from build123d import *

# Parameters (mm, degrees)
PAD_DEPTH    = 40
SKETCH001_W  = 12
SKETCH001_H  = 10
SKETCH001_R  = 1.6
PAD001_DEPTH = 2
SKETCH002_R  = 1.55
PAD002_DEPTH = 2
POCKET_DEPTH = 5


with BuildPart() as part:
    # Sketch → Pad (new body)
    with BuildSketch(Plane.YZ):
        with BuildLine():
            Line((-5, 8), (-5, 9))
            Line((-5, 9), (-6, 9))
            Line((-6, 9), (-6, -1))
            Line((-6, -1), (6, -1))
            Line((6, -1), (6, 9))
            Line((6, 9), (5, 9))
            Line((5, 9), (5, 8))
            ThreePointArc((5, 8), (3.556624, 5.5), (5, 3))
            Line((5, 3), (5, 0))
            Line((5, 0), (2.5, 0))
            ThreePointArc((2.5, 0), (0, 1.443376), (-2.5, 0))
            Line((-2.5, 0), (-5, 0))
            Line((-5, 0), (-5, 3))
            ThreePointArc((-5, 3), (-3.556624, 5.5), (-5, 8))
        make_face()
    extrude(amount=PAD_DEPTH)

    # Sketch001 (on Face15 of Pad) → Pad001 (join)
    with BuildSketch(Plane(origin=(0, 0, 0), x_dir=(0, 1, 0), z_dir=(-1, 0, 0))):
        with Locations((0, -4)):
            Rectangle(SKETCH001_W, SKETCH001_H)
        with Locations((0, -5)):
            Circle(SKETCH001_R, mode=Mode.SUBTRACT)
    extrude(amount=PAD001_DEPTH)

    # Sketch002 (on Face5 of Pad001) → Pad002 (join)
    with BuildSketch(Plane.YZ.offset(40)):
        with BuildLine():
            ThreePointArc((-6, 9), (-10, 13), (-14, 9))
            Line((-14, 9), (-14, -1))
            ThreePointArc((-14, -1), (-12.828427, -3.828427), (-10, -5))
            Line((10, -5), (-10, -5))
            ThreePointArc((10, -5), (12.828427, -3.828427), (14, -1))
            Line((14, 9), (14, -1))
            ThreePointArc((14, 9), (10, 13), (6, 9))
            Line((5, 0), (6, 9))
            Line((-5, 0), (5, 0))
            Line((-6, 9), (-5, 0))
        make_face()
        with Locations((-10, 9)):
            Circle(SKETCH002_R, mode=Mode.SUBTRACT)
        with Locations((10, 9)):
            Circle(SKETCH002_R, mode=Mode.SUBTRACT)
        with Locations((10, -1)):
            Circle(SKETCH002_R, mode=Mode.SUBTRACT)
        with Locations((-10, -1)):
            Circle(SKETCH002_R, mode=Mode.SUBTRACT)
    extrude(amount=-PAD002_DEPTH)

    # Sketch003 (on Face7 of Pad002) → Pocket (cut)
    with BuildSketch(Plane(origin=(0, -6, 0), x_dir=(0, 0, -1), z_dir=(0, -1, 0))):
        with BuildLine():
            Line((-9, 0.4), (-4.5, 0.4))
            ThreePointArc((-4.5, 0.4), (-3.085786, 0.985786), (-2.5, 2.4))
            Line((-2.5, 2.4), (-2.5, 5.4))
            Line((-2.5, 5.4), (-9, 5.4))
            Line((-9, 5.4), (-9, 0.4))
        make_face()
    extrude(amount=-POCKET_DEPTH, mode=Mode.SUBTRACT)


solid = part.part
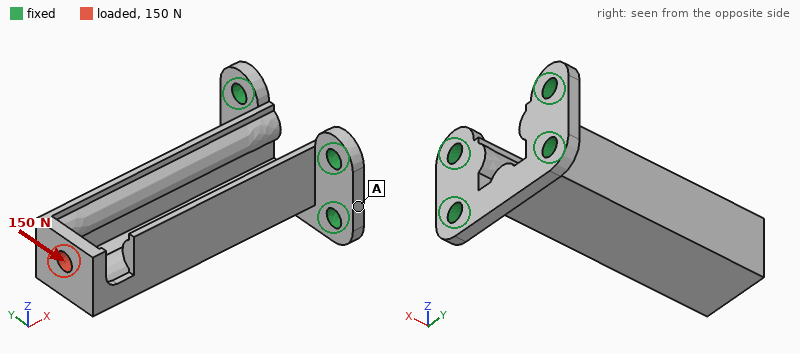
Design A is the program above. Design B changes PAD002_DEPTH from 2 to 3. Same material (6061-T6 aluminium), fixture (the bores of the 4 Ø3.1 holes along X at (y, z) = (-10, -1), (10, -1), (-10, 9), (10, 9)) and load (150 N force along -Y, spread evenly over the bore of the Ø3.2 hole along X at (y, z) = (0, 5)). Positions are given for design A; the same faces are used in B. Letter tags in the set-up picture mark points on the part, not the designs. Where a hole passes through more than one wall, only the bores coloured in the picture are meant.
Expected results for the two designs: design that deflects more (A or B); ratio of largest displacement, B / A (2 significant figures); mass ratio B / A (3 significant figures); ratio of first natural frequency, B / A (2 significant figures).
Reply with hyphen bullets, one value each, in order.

- A
- 0.86
- 1.11
- 1.1
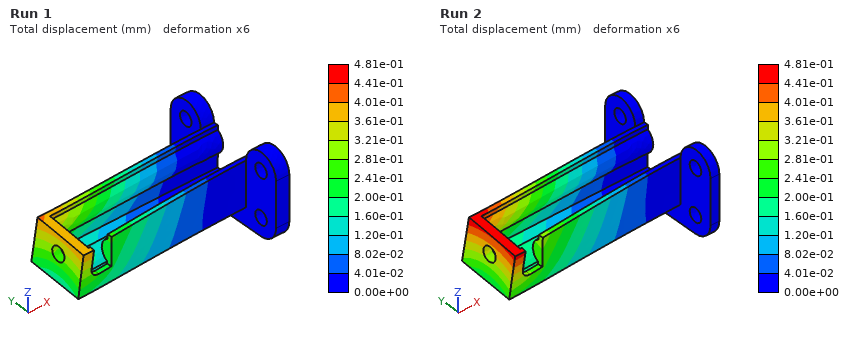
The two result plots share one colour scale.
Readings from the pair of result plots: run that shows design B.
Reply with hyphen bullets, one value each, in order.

- Run 1
